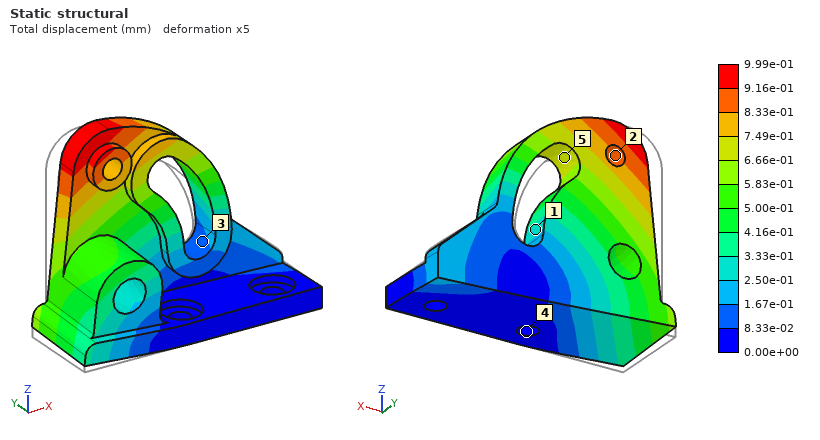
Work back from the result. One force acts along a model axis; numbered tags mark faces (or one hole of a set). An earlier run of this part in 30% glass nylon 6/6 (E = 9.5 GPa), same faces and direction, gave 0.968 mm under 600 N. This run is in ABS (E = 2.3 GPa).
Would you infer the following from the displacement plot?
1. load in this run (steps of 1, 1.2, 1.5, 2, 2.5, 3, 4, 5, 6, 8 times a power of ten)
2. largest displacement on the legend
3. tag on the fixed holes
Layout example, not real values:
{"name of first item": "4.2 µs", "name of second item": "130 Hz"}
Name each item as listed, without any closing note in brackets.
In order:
{"load in this run": "150 N", "largest displacement on the legend": "9.99e-01 mm", "tag on the fixed holes": "4"}
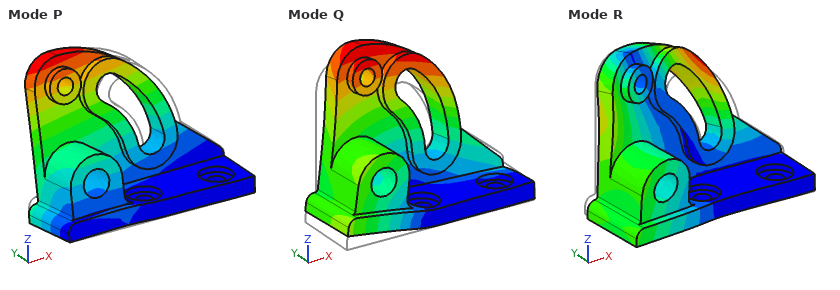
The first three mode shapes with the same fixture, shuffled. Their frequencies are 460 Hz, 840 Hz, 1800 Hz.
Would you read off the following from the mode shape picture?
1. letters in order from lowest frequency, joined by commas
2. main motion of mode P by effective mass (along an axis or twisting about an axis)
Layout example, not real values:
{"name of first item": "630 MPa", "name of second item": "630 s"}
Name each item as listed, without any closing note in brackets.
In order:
{"letters in order from lowest frequency, joined by commas": "P, Q, R", "main motion of mode P by effective mass": "along Y"}
